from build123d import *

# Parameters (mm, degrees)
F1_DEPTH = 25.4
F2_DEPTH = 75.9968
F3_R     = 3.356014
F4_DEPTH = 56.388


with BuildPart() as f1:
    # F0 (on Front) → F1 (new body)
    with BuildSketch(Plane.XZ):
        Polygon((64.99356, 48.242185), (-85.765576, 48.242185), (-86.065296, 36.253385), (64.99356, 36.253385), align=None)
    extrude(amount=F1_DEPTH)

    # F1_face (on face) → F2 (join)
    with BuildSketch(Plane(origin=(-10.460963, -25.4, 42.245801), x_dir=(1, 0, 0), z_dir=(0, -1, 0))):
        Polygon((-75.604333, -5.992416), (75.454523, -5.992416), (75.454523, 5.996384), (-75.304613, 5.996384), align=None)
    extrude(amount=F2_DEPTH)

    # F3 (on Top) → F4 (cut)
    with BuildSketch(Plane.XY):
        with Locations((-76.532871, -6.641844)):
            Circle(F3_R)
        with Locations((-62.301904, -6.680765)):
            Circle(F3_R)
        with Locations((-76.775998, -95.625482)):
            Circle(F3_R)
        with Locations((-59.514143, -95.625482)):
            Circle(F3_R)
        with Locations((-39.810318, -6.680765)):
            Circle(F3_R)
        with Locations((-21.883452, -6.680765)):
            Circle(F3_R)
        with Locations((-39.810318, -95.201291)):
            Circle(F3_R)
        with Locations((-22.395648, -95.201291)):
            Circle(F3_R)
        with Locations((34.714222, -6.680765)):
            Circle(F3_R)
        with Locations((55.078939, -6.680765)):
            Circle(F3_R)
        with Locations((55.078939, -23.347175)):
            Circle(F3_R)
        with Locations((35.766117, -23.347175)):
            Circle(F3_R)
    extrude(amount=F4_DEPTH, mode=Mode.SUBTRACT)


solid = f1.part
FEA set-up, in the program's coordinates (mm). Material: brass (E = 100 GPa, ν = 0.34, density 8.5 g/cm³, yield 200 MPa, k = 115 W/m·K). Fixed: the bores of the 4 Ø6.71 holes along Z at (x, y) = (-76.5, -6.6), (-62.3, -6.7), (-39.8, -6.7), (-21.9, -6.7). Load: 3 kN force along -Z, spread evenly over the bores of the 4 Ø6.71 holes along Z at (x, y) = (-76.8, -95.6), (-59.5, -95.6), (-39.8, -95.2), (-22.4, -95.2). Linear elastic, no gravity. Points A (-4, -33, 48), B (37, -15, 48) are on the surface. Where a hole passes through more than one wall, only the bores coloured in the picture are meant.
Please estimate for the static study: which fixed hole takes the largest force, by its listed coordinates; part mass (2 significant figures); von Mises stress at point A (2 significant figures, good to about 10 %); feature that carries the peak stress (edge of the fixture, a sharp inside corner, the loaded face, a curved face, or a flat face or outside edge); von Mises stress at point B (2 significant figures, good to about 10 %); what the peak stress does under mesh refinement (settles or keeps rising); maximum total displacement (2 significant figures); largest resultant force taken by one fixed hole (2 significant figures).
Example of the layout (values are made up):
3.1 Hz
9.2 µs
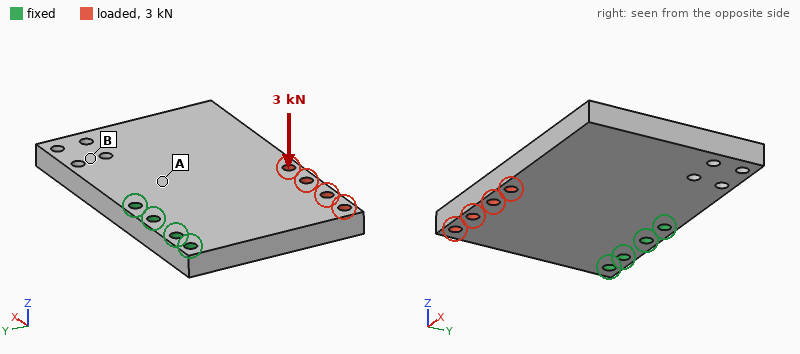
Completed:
(-39.8, -6.7)
1.5 kg
47 MPa
edge of the fixture
15 MPa
keeps rising
0.56 mm
1.5 kN
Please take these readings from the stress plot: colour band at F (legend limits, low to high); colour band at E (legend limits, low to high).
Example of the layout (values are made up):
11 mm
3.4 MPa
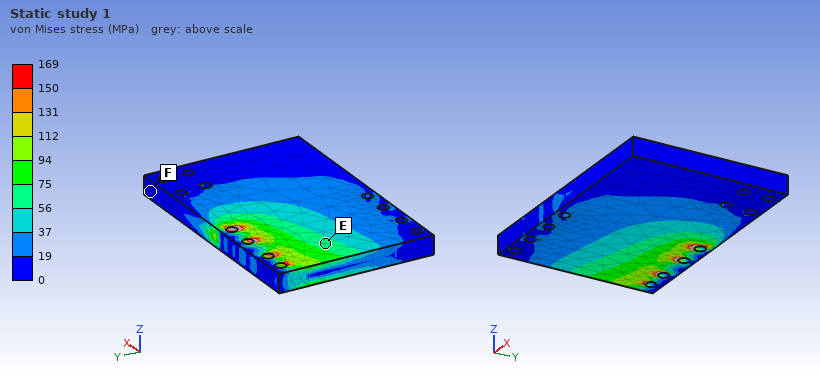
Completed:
0 to 19 MPa
56 to 75 MPa
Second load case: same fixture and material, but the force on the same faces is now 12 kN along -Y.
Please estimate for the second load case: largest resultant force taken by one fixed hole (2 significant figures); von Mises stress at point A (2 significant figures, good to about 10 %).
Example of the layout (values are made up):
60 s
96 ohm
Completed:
3.3 kN
4.4 MPa
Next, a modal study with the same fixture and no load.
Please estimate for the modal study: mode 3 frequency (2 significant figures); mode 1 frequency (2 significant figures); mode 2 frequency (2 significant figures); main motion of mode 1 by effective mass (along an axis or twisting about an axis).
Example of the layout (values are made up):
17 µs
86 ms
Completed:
1600 Hz
470 Hz
830 Hz
along Z
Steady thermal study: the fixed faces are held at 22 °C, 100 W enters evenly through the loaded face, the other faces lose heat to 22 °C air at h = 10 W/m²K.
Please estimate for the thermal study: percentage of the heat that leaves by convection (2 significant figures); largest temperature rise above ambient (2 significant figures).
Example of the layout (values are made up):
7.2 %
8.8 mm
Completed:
11 %
75 K
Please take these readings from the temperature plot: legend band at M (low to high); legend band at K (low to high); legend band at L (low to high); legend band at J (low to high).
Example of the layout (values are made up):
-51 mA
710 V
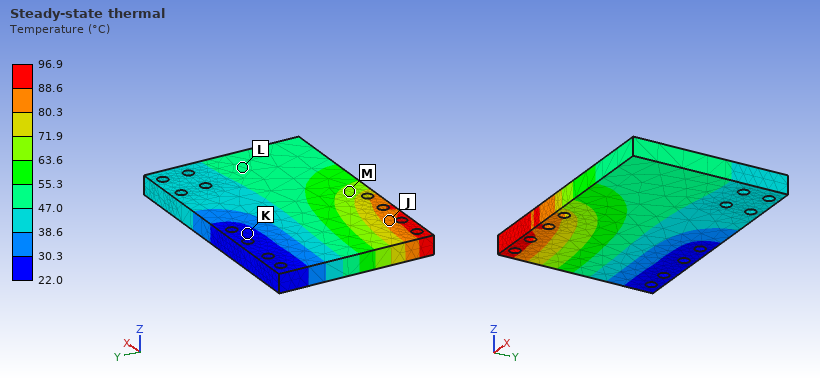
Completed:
63.6 to 71.9 °C
22.0 to 30.3 °C
47.0 to 55.3 °C
80.3 to 88.6 °C
